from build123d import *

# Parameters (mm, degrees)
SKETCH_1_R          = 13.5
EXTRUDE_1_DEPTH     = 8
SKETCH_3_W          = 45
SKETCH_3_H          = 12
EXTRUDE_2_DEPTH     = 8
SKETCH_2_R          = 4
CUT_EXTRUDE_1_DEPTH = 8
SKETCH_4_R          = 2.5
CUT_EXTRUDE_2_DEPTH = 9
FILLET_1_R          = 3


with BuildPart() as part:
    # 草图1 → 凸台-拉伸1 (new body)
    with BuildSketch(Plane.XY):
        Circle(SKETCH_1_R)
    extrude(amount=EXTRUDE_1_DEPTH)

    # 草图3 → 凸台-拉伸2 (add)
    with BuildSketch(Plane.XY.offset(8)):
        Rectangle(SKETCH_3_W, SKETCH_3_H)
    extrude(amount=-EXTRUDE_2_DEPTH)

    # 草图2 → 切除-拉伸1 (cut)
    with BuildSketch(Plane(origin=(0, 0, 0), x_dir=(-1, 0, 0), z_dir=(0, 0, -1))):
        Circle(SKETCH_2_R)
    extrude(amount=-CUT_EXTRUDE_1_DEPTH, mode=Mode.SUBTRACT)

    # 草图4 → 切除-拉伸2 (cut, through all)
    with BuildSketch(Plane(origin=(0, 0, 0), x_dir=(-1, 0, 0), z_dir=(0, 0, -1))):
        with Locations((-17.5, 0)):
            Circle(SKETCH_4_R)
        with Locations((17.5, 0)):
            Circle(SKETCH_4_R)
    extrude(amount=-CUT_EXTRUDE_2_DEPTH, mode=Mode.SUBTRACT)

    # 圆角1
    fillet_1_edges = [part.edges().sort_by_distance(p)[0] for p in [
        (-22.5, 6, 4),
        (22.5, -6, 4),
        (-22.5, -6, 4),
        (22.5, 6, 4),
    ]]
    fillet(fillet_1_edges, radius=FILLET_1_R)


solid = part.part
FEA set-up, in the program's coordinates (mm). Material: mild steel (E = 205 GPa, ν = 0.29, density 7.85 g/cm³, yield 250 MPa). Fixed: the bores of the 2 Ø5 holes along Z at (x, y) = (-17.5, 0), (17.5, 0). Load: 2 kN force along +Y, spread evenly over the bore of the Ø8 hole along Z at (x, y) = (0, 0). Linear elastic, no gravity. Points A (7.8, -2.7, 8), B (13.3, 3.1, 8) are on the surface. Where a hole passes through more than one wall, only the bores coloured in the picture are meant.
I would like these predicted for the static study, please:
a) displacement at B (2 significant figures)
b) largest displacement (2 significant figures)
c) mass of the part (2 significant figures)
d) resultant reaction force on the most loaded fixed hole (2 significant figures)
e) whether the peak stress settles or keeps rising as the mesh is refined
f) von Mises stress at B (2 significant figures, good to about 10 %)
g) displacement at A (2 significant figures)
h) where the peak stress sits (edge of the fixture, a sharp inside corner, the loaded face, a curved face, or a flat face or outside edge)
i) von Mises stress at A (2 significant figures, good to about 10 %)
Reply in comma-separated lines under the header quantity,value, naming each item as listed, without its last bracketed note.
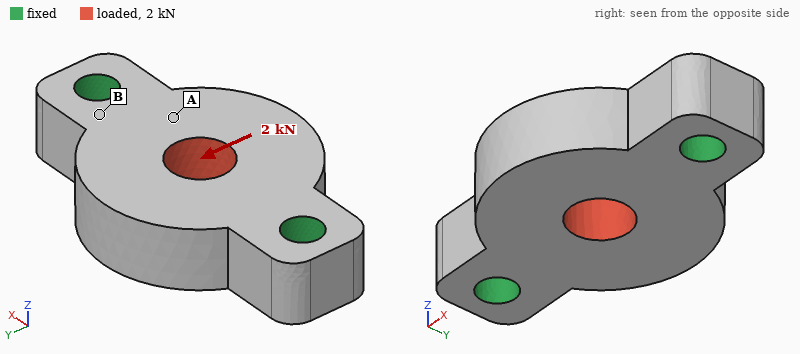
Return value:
quantity,value
displacement at B,0.58 µm
largest displacement,2.0 µm
mass of the part,44 g
resultant reaction force on the most loaded fixed hole,1.0 kN
whether the peak stress settles or keeps rising as the mesh is refined,keeps rising
von Mises stress at B,21 MPa
displacement at A,1.4 µm
where the peak stress sits,edge of the fixture
von Mises stress at A,9.0 MPa
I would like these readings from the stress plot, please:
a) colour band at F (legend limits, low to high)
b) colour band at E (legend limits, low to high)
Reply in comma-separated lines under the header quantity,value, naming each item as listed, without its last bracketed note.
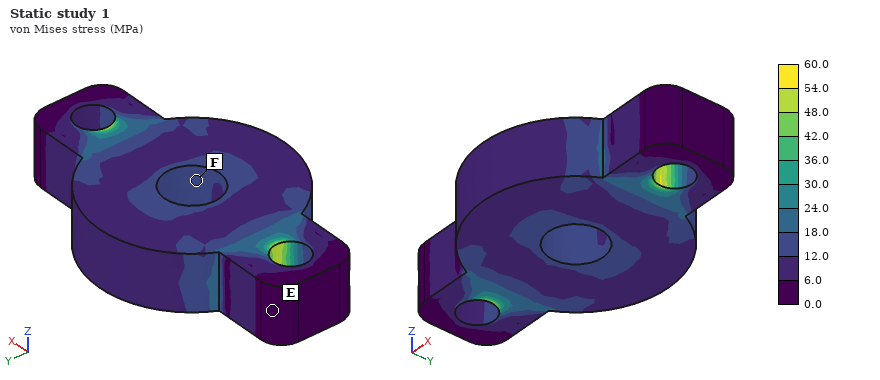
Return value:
quantity,value
colour band at F,12.0 to 18.0 MPa
colour band at E,0.0 to 6.0 MPa
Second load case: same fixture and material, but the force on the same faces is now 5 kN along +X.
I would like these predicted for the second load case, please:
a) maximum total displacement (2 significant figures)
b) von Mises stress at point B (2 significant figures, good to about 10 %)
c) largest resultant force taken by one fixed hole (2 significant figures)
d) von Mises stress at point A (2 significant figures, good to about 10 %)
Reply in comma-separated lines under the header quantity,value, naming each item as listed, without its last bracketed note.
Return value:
quantity,value
maximum total displacement,2.0 µm
von Mises stress at point B,23 MPa
largest resultant force taken by one fixed hole,2.5 kN
von Mises stress at point A,28 MPa
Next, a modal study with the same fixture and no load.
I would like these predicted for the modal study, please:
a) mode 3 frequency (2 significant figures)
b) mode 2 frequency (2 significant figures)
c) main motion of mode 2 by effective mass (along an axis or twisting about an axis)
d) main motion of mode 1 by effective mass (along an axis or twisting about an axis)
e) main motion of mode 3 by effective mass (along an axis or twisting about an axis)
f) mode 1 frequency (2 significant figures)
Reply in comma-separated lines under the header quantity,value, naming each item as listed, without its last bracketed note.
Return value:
quantity,value
mode 3 frequency,34 kHz
mode 2 frequency,22 kHz
main motion of mode 2 by effective mass,along Z
main motion of mode 1 by effective mass,twisting about X
main motion of mode 3 by effective mass,along Y
mode 1 frequency,19 kHz
